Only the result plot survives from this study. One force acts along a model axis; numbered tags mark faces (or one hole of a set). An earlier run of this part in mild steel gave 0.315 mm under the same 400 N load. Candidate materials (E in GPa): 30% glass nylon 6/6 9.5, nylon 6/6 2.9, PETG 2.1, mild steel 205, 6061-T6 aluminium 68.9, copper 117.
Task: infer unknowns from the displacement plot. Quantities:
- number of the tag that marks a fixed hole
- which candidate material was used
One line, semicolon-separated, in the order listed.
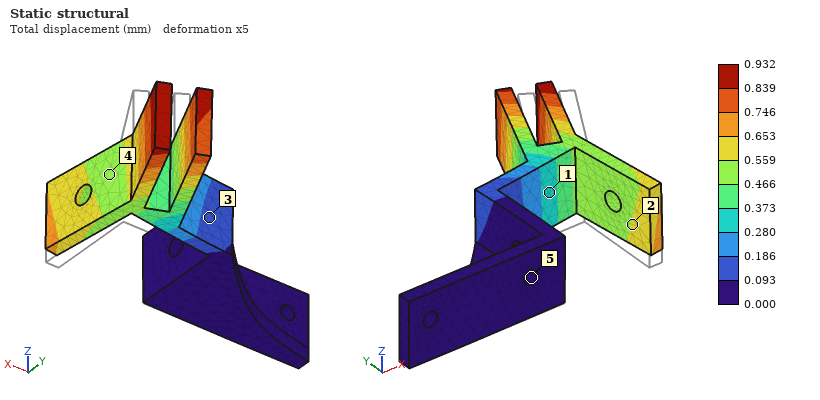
5; 6061-T6 aluminium
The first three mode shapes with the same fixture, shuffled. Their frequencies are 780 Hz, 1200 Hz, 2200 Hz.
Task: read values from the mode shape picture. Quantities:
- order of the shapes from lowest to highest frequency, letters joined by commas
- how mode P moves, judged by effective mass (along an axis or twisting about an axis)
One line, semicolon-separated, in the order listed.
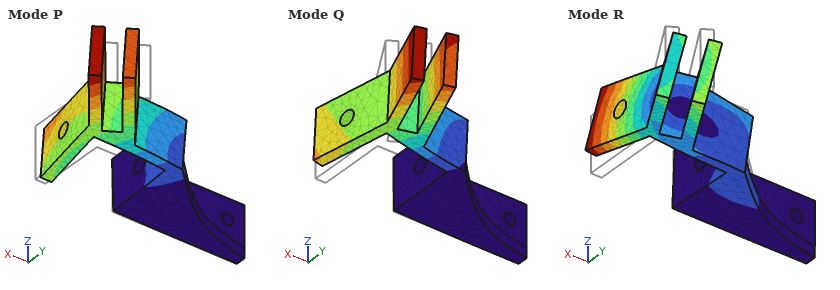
Q, P, R; along Z
